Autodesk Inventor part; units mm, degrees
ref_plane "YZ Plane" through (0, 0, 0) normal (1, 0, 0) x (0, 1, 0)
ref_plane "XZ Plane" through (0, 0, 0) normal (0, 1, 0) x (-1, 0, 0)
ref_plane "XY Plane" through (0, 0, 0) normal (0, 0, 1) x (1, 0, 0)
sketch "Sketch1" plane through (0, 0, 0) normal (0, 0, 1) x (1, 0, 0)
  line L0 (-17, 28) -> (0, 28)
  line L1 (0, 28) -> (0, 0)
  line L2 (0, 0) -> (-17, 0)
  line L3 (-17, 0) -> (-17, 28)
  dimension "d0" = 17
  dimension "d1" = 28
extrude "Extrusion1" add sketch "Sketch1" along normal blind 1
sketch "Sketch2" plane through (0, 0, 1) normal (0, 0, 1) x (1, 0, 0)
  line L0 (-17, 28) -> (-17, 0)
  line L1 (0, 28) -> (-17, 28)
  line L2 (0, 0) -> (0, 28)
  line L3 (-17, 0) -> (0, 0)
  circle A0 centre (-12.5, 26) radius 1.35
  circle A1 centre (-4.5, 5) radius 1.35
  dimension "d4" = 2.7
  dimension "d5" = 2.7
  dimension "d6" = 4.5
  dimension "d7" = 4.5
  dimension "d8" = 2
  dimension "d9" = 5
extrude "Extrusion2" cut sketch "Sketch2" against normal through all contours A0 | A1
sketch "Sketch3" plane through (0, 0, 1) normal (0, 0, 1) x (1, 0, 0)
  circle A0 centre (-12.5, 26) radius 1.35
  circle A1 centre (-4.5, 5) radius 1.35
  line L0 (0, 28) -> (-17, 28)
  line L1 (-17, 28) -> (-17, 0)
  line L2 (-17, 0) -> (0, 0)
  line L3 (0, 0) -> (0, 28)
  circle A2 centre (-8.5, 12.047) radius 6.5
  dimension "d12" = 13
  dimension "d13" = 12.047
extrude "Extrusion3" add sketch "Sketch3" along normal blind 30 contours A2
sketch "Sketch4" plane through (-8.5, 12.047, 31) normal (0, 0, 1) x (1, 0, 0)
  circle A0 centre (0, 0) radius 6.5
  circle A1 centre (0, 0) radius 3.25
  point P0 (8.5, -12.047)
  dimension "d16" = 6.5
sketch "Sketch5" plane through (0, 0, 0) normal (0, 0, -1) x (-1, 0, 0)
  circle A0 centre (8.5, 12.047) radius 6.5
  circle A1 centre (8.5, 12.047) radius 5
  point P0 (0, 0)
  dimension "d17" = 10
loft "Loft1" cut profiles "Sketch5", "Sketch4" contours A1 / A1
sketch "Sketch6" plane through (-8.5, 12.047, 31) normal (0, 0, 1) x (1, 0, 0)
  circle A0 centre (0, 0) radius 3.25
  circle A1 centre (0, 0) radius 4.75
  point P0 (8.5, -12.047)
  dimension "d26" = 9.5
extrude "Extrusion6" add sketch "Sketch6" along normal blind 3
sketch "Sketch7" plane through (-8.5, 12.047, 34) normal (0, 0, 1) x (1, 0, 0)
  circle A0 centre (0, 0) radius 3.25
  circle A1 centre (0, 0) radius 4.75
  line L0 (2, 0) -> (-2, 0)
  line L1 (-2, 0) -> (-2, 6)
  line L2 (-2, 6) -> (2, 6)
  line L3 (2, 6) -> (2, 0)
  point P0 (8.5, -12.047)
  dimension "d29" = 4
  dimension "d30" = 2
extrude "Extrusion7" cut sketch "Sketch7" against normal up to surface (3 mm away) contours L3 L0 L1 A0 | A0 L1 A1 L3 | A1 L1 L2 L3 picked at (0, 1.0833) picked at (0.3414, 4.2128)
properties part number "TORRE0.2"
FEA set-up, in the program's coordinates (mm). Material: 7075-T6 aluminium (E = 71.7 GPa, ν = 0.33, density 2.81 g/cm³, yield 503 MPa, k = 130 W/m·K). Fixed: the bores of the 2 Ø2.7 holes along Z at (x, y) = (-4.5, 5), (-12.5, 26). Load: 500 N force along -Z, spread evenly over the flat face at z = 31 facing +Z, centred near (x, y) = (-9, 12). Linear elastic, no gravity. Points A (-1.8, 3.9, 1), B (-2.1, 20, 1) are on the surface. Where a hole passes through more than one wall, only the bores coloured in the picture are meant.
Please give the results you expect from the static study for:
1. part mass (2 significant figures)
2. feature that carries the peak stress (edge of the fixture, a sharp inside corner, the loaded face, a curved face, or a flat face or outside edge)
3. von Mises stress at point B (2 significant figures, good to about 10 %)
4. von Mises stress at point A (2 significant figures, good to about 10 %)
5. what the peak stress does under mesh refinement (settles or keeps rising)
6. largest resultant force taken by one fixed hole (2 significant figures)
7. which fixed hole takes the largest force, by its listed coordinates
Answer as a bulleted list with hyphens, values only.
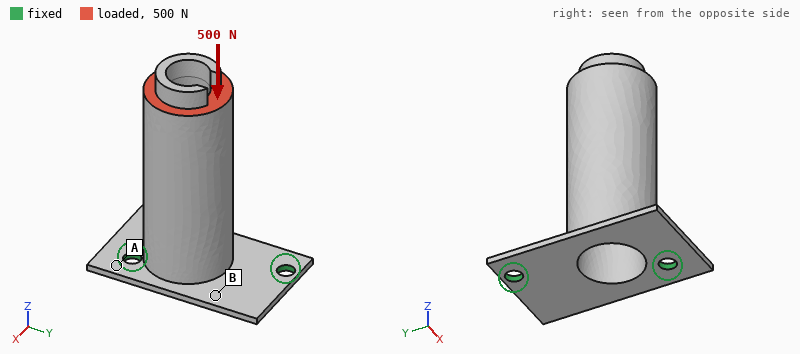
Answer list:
- 8.0 g
- edge of the fixture
- 83 MPa
- 31 MPa
- keeps rising
- 320 N
- (-4.5, 5)
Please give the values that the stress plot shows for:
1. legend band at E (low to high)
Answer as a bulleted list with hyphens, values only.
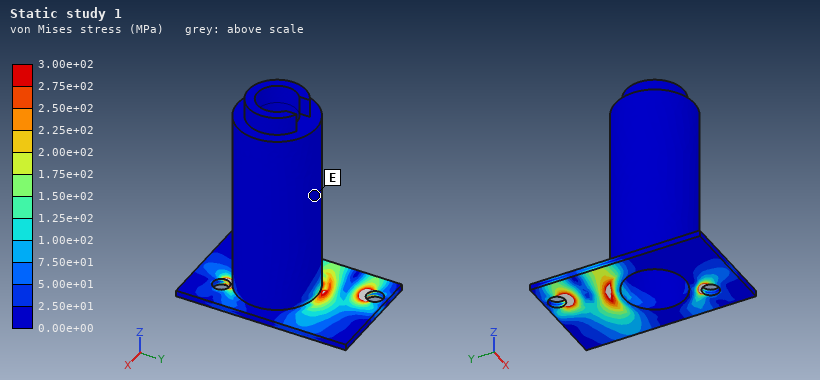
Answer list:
- 0.00e+00 to 2.50e+01 MPa
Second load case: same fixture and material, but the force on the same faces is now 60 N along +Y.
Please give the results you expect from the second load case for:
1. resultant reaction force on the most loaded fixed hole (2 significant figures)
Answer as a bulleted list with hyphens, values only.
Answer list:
- 95 N
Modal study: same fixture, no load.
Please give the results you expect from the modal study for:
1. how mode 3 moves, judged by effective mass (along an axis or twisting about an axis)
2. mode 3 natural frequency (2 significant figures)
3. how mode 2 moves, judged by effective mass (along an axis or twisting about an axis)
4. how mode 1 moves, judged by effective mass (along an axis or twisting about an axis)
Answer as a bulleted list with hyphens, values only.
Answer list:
- along Z
- 11 kHz
- along Y
- along X
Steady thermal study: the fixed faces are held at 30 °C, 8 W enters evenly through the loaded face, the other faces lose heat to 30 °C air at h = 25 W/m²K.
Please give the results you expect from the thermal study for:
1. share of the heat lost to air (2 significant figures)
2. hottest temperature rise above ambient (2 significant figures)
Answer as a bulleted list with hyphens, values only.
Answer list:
- 18 %
- 33 K
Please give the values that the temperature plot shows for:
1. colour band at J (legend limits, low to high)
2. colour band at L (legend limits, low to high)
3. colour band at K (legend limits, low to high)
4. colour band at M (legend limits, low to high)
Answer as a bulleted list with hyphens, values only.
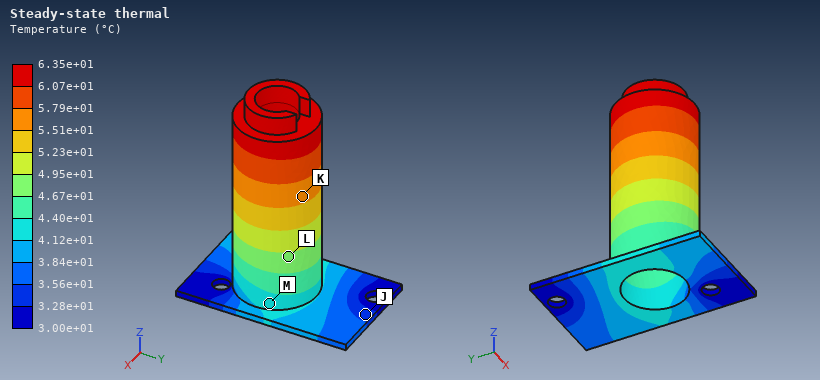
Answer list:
- 3.28e+01 to 3.56e+01 °C
- 4.67e+01 to 4.95e+01 °C
- 5.51e+01 to 5.79e+01 °C
- 4.12e+01 to 4.40e+01 °C
